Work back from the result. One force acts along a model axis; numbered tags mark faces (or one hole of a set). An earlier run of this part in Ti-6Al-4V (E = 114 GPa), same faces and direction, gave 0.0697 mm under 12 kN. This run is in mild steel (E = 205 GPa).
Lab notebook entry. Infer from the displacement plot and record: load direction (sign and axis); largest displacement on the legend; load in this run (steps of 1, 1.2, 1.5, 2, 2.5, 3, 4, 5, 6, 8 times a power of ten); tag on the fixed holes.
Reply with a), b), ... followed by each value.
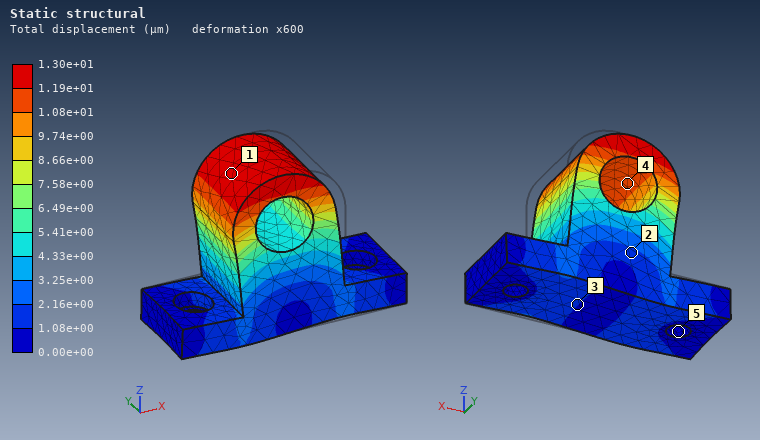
a) -X
b) 1.30e+01 µm
c) 4 kN
d) 5
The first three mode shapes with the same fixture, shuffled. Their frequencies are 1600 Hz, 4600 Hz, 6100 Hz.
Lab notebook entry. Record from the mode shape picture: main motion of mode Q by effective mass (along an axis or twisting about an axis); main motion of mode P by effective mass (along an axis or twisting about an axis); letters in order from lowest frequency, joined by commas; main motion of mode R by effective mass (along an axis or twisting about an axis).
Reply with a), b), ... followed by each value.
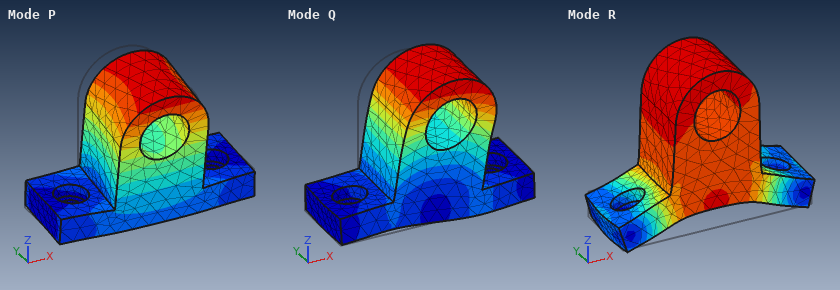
a) along X
b) along Y
c) P, Q, R
d) along Z
